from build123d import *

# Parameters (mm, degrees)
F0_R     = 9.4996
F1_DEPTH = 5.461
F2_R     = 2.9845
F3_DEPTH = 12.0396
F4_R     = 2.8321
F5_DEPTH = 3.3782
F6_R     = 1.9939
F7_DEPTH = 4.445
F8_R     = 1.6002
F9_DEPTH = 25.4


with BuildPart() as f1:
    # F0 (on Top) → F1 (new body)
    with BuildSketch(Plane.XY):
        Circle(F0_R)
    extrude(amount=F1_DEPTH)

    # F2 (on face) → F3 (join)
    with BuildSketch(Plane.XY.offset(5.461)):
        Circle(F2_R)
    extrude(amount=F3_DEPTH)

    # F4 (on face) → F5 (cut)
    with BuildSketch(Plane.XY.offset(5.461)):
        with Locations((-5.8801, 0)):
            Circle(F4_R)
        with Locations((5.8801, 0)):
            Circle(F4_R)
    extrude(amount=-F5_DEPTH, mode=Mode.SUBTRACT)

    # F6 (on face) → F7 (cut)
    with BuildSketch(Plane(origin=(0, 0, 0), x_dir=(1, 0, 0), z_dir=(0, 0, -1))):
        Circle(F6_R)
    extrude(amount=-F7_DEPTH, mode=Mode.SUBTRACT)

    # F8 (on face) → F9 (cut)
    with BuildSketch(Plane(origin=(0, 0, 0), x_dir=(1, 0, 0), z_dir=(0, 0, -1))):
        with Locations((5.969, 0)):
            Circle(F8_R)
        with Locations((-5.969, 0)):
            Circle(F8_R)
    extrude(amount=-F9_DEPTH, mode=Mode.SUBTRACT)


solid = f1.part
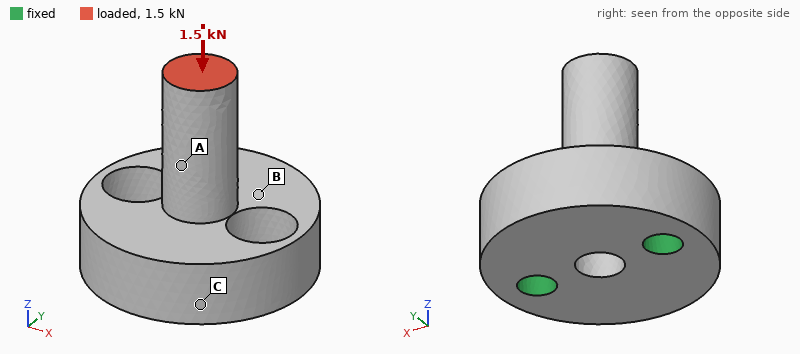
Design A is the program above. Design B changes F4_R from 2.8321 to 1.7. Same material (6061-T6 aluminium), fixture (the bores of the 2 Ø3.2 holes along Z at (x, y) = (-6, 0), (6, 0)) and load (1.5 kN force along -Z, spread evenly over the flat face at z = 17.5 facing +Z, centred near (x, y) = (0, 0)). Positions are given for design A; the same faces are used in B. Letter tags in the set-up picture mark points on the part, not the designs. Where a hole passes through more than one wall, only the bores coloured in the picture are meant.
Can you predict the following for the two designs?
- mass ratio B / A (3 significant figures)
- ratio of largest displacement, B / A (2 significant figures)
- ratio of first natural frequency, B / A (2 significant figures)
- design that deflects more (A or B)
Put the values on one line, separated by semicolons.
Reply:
1.07; 0.85; 1.1; A
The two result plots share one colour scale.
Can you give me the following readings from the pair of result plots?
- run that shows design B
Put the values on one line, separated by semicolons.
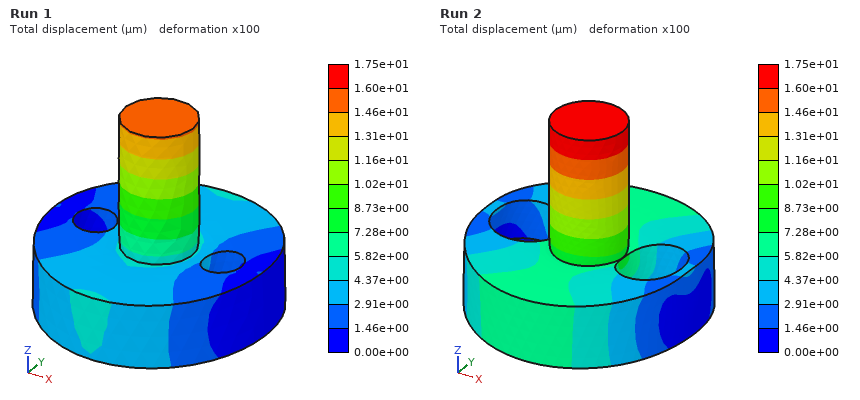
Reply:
Run 1
